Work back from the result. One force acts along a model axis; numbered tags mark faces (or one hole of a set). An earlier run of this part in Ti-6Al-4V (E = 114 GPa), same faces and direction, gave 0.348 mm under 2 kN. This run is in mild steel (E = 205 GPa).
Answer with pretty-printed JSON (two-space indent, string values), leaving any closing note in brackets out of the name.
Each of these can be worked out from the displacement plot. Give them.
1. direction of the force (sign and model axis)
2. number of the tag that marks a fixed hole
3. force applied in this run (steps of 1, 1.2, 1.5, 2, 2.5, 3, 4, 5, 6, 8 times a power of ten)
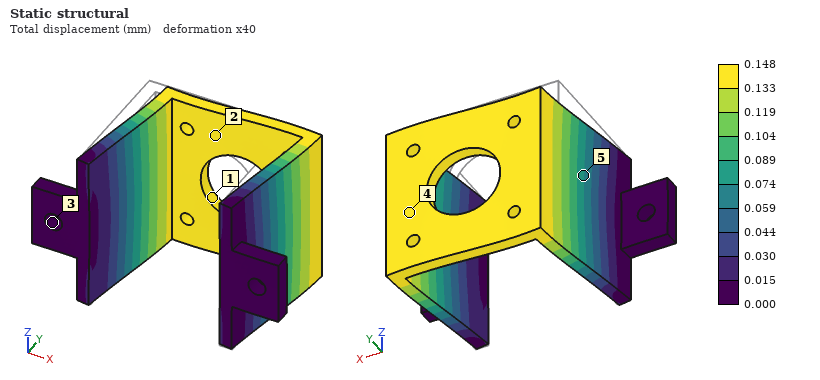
{
  "direction of the force": "+X",
  "number of the tag that marks a fixed hole": "3",
  "force applied in this run": "1.5 kN"
}
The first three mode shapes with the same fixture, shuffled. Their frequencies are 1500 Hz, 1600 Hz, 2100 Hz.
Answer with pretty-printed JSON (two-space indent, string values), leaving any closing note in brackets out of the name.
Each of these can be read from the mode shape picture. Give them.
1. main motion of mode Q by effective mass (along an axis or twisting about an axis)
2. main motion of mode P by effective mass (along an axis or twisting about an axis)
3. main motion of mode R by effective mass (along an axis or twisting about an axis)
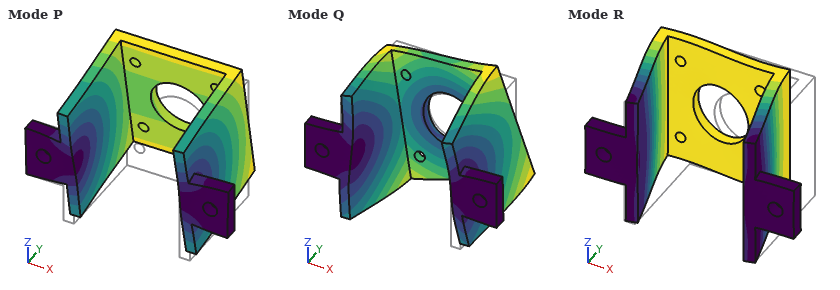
{
  "main motion of mode Q by effective mass": "twisting about Y",
  "main motion of mode P by effective mass": "along Z",
  "main motion of mode R by effective mass": "along X"
}
